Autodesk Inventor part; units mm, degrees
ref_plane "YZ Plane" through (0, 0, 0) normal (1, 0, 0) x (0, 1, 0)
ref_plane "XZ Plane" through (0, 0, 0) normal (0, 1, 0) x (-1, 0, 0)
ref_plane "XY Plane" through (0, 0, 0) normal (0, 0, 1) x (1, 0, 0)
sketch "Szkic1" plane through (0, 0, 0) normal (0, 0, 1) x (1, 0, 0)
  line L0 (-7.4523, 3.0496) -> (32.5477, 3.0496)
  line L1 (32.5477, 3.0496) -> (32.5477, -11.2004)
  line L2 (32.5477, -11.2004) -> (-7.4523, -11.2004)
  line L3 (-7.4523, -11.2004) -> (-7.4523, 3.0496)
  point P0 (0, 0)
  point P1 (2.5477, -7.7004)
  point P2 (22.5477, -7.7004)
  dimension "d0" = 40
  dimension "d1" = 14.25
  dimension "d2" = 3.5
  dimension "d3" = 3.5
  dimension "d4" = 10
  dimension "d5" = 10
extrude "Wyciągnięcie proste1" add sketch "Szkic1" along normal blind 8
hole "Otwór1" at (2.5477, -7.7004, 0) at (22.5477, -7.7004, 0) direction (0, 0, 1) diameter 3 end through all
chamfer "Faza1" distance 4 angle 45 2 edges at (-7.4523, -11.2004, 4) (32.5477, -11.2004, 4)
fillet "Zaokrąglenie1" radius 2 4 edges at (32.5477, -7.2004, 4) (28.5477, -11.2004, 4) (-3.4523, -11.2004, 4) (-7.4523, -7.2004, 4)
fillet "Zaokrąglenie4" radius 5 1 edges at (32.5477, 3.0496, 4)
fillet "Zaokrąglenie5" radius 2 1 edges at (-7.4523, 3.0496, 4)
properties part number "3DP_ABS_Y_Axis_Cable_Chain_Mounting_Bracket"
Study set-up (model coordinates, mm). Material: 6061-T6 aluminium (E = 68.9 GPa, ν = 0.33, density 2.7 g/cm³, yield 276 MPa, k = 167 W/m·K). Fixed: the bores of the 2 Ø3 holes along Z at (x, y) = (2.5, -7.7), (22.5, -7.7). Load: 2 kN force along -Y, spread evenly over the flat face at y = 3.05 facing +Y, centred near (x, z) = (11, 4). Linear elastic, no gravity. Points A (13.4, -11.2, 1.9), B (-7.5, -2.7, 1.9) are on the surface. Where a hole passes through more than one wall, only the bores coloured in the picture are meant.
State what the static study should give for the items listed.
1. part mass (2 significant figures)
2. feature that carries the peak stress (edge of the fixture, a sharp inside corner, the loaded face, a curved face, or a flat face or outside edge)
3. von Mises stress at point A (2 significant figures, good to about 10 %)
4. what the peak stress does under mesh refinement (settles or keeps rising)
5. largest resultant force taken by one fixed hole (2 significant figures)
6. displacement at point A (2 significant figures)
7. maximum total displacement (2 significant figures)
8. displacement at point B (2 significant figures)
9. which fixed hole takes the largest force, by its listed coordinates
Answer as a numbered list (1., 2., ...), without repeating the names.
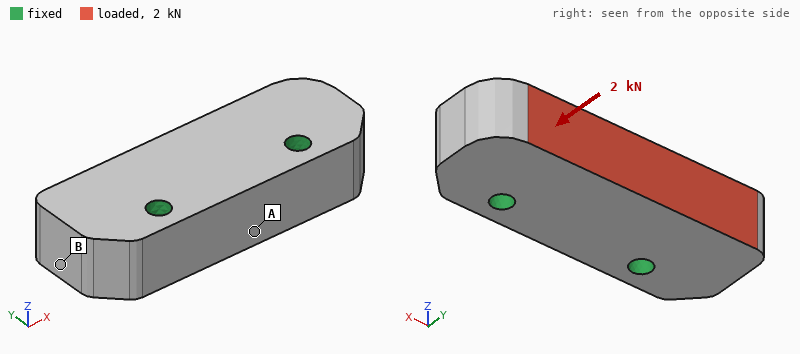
1. 12 g
2. edge of the fixture
3. 6.3 MPa
4. keeps rising
5. 1.1 kN
6. 1.4 µm
7. 2.4 µm
8. 2.1 µm
9. (2.5, -7.7)
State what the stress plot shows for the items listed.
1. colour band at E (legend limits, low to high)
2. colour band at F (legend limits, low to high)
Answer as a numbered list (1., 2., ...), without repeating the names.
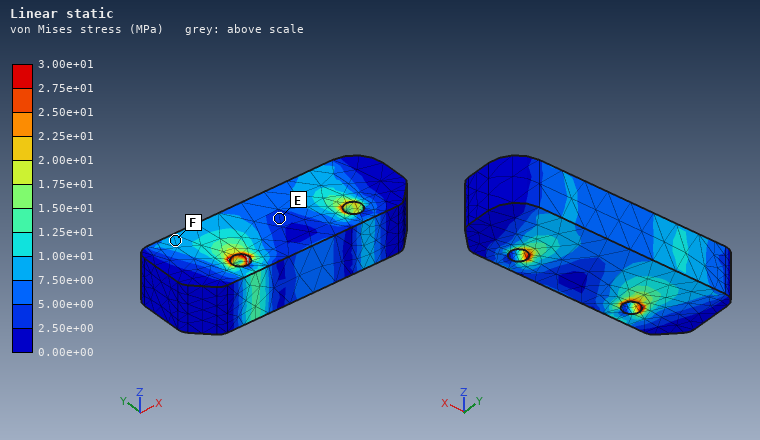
1. 2.50e+00 to 5.00e+00 MPa
2. 7.50e+00 to 1.00e+01 MPa
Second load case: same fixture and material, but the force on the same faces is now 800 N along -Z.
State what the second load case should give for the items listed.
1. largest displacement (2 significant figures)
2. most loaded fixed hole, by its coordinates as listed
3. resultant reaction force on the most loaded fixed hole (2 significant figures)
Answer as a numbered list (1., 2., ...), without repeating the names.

1. 8.4 µm
2. (2.5, -7.7)
3. 440 N
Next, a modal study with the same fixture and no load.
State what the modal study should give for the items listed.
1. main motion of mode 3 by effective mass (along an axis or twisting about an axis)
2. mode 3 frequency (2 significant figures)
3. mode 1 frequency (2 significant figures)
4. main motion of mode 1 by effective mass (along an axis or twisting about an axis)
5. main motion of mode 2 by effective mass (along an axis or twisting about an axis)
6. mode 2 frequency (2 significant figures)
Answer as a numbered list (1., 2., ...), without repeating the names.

1. along X
2. 39 kHz
3. 31 kHz
4. along Z
5. twisting about Y
6. 35 kHz
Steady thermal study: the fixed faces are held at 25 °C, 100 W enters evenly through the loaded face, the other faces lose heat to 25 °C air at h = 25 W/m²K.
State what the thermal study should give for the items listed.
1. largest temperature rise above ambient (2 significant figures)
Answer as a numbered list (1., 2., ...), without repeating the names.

1. 29 K
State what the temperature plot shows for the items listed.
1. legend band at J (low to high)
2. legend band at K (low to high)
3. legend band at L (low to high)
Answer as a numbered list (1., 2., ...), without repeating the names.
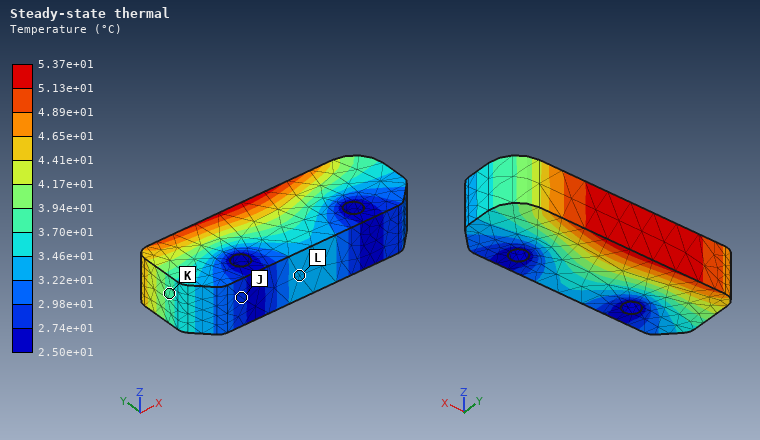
1. 2.74e+01 to 2.98e+01 °C
2. 3.70e+01 to 3.94e+01 °C
3. 3.22e+01 to 3.46e+01 °C
